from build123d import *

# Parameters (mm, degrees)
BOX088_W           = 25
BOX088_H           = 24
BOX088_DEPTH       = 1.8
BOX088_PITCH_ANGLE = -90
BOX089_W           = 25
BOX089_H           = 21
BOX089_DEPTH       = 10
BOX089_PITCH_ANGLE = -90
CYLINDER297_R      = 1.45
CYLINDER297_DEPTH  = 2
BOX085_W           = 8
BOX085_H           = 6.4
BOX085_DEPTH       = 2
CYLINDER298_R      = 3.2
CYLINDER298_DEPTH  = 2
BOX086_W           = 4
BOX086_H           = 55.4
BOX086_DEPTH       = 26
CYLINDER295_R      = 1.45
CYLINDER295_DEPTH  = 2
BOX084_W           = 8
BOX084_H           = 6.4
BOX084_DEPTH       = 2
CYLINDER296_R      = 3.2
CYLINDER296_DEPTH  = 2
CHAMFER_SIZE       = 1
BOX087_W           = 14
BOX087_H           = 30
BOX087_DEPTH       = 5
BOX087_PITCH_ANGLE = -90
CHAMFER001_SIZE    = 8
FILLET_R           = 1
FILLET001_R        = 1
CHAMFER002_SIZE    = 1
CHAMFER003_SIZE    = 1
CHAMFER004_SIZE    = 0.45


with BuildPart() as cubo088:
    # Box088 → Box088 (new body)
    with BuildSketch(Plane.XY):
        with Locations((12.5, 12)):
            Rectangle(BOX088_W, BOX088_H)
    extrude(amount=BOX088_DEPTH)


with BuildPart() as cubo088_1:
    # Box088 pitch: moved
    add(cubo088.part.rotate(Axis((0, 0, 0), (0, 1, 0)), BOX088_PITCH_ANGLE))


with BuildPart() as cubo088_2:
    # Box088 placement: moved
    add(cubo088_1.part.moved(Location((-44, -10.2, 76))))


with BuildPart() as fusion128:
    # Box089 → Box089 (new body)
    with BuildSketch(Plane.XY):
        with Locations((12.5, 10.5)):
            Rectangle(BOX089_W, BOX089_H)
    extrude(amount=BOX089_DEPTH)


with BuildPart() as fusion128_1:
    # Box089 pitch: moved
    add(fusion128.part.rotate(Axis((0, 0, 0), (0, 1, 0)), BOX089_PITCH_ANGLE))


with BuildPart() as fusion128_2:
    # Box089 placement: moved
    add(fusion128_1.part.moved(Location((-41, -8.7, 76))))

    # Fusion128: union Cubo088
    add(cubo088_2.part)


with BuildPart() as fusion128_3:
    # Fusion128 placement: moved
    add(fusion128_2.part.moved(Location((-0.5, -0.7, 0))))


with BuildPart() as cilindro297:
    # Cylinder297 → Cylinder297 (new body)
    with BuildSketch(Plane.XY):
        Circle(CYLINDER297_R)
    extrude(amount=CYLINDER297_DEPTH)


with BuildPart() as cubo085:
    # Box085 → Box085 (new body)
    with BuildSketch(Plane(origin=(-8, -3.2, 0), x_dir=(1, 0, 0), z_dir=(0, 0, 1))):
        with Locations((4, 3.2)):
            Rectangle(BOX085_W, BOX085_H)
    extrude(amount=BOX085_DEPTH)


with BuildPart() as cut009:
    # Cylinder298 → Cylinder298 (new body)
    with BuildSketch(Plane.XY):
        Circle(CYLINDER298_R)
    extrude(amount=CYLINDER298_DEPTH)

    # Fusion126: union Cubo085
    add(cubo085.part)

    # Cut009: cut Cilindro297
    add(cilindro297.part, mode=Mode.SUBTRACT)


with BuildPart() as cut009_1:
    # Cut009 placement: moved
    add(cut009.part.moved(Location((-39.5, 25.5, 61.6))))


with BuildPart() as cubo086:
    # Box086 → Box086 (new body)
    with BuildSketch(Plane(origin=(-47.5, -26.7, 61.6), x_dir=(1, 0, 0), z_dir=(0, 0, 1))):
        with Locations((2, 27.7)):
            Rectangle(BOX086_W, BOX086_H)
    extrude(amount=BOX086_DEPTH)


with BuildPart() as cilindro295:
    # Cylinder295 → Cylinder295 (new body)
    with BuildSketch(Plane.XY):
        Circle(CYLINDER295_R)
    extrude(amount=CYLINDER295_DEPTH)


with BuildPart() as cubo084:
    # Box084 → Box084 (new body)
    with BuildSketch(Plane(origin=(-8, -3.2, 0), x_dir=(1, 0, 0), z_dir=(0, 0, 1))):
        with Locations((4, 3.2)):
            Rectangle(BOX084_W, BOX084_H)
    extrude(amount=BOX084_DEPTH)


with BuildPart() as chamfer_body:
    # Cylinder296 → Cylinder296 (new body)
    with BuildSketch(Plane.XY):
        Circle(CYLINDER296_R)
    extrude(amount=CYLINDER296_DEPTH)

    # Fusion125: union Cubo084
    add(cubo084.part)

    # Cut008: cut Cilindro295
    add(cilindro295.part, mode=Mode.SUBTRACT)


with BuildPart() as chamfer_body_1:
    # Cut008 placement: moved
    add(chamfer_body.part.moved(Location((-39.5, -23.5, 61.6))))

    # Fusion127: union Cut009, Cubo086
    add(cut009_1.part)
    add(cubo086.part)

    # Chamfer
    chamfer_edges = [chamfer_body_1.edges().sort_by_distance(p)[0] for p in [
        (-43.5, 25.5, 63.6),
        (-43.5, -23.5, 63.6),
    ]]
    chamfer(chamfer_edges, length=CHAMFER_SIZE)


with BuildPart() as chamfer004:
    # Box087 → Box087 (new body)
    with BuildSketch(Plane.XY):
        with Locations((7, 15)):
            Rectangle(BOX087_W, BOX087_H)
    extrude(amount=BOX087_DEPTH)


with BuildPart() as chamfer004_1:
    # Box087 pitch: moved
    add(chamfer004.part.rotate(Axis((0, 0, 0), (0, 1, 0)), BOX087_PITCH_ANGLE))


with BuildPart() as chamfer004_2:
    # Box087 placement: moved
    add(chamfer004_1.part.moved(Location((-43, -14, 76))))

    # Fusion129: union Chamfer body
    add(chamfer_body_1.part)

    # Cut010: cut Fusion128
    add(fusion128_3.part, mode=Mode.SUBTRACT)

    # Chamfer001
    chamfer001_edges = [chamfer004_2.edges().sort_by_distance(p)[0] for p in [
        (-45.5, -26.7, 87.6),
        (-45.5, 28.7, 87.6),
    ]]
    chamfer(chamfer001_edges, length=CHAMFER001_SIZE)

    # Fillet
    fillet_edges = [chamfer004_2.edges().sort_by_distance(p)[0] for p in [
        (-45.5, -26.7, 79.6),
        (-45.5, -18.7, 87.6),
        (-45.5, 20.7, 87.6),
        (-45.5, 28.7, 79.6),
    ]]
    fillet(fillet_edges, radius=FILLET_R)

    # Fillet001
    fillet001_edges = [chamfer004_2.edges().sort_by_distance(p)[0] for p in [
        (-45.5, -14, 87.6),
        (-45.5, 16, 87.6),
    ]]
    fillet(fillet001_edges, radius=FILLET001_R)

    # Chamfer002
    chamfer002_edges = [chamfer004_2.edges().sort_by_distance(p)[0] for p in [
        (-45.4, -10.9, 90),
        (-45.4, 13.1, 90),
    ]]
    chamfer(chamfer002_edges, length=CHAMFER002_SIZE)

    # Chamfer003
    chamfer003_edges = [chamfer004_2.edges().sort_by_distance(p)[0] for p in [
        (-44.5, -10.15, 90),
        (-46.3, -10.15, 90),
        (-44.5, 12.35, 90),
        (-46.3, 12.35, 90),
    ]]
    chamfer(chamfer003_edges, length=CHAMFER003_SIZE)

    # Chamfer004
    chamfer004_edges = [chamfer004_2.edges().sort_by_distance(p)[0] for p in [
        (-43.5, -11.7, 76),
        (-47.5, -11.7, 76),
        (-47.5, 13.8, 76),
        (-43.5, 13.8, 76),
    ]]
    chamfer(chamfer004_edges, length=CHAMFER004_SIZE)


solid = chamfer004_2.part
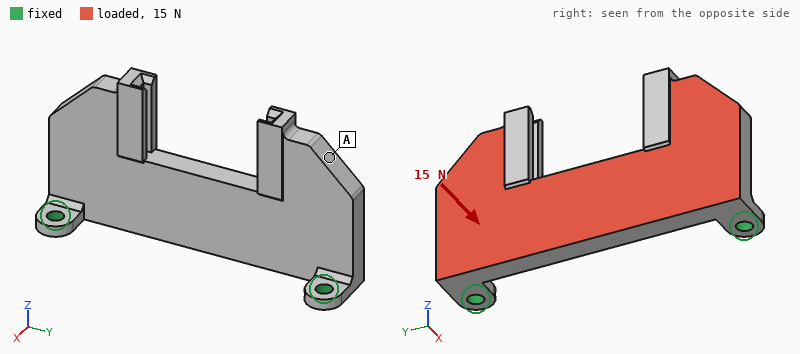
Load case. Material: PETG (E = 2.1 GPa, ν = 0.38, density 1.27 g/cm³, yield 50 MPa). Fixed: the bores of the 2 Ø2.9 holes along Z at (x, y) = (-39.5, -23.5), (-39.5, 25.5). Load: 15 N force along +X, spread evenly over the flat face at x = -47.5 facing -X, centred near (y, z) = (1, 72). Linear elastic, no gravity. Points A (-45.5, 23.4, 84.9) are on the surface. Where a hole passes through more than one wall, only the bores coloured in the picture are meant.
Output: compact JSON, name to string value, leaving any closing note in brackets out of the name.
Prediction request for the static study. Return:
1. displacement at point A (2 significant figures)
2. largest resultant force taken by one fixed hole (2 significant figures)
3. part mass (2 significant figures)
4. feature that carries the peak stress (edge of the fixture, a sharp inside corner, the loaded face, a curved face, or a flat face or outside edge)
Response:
{"displacement at point A": "0.56 mm", "largest resultant force taken by one fixed hole": "8.8 N", "part mass": "6.1 g", "feature that carries the peak stress": "a flat face or outside edge"}
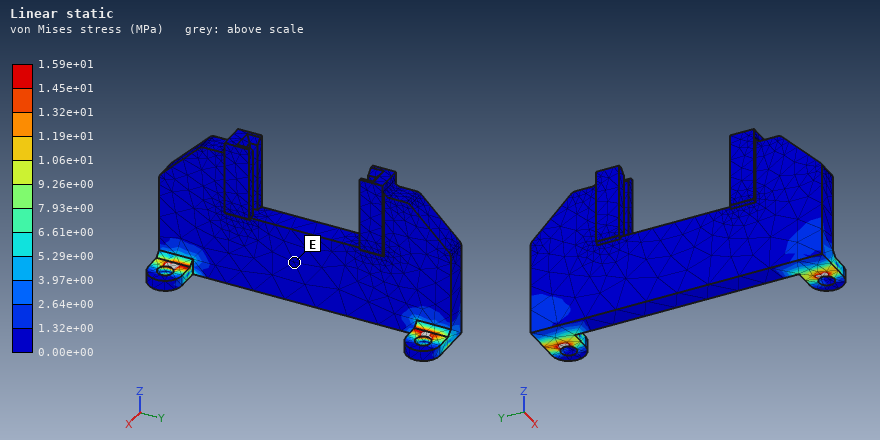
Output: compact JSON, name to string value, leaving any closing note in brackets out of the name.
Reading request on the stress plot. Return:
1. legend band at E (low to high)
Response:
{"legend band at E": "0.00e+00 to 1.32e+00 MPa"}
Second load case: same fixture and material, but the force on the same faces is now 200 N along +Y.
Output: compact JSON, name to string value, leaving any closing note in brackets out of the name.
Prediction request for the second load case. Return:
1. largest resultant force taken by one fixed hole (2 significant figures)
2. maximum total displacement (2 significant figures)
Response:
{"largest resultant force taken by one fixed hole": "110 N", "maximum total displacement": "0.23 mm"}
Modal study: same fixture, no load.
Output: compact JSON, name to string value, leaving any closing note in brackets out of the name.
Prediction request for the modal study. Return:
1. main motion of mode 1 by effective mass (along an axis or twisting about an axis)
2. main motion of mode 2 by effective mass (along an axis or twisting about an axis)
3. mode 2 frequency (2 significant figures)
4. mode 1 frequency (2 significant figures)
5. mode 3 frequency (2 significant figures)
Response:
{"main motion of mode 1 by effective mass": "along X", "main motion of mode 2 by effective mass": "twisting about Z", "mode 2 frequency": "970 Hz", "mode 1 frequency": "360 Hz", "mode 3 frequency": "1800 Hz"}
